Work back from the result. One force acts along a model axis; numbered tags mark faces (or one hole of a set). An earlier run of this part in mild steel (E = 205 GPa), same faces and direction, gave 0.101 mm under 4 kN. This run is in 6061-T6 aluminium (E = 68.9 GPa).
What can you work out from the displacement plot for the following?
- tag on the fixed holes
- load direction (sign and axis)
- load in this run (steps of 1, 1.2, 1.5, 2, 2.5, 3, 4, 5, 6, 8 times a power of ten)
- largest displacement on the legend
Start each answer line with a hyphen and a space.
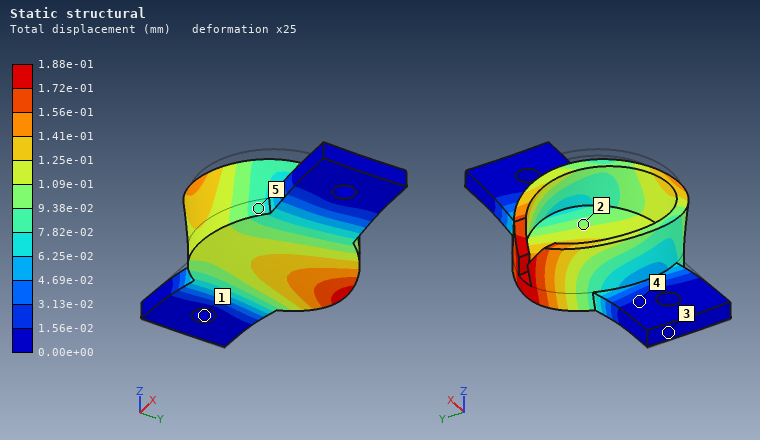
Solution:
- 1
- -Z
- 2.5 kN
- 1.88e-01 mm
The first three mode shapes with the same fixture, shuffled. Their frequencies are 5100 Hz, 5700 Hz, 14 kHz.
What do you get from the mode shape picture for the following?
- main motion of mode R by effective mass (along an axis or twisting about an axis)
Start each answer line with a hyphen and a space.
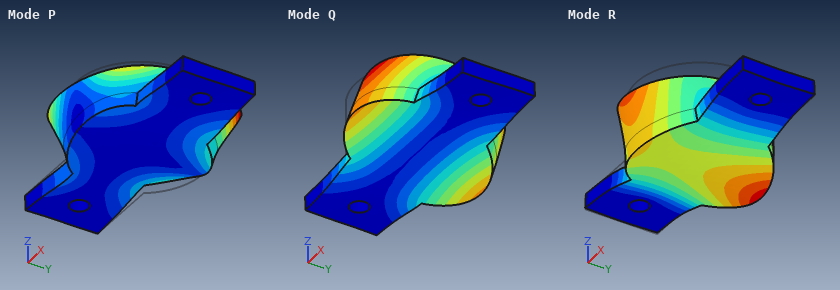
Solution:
- along Z
